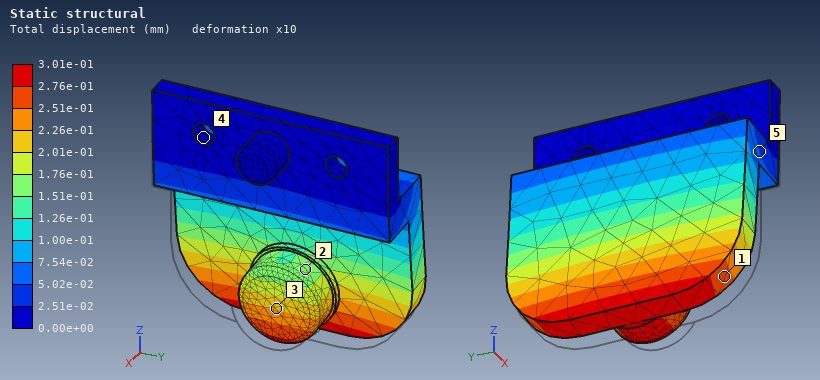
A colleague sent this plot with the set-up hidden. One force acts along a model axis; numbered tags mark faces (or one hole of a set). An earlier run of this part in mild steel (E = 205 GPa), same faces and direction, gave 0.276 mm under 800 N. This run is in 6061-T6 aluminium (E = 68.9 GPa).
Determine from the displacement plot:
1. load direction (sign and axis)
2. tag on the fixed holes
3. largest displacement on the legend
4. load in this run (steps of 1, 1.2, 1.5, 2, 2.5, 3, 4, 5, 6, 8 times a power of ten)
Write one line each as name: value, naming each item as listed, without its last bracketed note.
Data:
load direction: -X
tag on the fixed holes: 4
largest displacement on the legend: 3.01e-01 mm
load in this run: 300 N
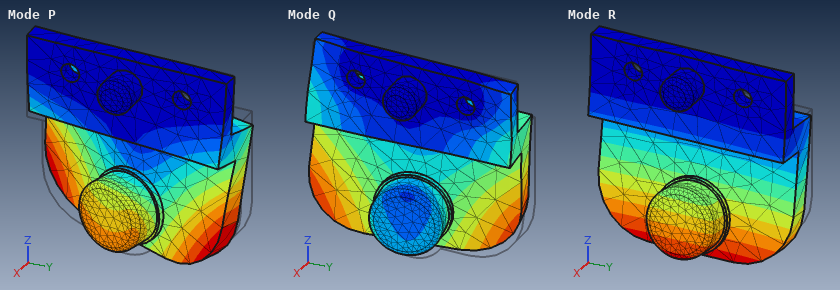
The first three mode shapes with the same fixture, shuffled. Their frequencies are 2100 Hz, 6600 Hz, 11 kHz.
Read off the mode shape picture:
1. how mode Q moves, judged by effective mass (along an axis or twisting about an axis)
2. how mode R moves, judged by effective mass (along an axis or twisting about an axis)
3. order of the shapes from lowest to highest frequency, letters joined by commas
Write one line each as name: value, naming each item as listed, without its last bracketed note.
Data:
how mode Q moves, judged by effective mass: along Y
how mode R moves, judged by effective mass: along X
order of the shapes from lowest to highest frequency, letters joined by commas: R, P, Q
